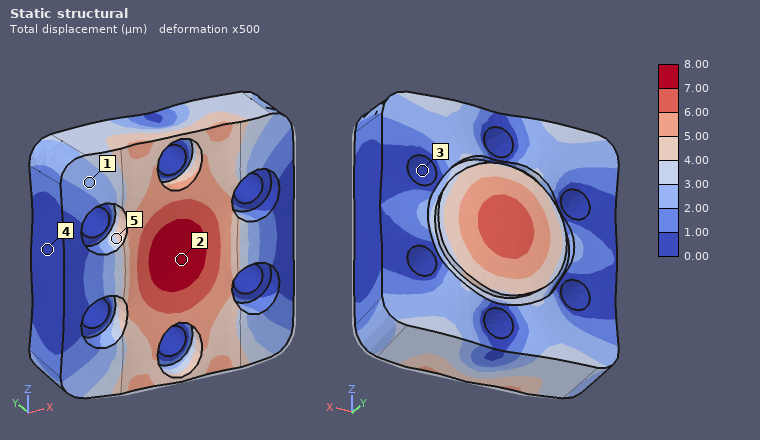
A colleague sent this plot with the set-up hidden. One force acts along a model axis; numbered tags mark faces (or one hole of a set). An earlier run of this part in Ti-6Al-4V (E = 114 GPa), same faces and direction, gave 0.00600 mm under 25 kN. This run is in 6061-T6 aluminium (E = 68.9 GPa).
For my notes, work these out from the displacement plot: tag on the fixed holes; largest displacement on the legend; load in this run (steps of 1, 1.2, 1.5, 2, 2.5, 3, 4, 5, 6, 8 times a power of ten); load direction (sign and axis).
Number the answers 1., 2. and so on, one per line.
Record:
1. 3
2. 8.00 µm
3. 20 kN
4. +Y
